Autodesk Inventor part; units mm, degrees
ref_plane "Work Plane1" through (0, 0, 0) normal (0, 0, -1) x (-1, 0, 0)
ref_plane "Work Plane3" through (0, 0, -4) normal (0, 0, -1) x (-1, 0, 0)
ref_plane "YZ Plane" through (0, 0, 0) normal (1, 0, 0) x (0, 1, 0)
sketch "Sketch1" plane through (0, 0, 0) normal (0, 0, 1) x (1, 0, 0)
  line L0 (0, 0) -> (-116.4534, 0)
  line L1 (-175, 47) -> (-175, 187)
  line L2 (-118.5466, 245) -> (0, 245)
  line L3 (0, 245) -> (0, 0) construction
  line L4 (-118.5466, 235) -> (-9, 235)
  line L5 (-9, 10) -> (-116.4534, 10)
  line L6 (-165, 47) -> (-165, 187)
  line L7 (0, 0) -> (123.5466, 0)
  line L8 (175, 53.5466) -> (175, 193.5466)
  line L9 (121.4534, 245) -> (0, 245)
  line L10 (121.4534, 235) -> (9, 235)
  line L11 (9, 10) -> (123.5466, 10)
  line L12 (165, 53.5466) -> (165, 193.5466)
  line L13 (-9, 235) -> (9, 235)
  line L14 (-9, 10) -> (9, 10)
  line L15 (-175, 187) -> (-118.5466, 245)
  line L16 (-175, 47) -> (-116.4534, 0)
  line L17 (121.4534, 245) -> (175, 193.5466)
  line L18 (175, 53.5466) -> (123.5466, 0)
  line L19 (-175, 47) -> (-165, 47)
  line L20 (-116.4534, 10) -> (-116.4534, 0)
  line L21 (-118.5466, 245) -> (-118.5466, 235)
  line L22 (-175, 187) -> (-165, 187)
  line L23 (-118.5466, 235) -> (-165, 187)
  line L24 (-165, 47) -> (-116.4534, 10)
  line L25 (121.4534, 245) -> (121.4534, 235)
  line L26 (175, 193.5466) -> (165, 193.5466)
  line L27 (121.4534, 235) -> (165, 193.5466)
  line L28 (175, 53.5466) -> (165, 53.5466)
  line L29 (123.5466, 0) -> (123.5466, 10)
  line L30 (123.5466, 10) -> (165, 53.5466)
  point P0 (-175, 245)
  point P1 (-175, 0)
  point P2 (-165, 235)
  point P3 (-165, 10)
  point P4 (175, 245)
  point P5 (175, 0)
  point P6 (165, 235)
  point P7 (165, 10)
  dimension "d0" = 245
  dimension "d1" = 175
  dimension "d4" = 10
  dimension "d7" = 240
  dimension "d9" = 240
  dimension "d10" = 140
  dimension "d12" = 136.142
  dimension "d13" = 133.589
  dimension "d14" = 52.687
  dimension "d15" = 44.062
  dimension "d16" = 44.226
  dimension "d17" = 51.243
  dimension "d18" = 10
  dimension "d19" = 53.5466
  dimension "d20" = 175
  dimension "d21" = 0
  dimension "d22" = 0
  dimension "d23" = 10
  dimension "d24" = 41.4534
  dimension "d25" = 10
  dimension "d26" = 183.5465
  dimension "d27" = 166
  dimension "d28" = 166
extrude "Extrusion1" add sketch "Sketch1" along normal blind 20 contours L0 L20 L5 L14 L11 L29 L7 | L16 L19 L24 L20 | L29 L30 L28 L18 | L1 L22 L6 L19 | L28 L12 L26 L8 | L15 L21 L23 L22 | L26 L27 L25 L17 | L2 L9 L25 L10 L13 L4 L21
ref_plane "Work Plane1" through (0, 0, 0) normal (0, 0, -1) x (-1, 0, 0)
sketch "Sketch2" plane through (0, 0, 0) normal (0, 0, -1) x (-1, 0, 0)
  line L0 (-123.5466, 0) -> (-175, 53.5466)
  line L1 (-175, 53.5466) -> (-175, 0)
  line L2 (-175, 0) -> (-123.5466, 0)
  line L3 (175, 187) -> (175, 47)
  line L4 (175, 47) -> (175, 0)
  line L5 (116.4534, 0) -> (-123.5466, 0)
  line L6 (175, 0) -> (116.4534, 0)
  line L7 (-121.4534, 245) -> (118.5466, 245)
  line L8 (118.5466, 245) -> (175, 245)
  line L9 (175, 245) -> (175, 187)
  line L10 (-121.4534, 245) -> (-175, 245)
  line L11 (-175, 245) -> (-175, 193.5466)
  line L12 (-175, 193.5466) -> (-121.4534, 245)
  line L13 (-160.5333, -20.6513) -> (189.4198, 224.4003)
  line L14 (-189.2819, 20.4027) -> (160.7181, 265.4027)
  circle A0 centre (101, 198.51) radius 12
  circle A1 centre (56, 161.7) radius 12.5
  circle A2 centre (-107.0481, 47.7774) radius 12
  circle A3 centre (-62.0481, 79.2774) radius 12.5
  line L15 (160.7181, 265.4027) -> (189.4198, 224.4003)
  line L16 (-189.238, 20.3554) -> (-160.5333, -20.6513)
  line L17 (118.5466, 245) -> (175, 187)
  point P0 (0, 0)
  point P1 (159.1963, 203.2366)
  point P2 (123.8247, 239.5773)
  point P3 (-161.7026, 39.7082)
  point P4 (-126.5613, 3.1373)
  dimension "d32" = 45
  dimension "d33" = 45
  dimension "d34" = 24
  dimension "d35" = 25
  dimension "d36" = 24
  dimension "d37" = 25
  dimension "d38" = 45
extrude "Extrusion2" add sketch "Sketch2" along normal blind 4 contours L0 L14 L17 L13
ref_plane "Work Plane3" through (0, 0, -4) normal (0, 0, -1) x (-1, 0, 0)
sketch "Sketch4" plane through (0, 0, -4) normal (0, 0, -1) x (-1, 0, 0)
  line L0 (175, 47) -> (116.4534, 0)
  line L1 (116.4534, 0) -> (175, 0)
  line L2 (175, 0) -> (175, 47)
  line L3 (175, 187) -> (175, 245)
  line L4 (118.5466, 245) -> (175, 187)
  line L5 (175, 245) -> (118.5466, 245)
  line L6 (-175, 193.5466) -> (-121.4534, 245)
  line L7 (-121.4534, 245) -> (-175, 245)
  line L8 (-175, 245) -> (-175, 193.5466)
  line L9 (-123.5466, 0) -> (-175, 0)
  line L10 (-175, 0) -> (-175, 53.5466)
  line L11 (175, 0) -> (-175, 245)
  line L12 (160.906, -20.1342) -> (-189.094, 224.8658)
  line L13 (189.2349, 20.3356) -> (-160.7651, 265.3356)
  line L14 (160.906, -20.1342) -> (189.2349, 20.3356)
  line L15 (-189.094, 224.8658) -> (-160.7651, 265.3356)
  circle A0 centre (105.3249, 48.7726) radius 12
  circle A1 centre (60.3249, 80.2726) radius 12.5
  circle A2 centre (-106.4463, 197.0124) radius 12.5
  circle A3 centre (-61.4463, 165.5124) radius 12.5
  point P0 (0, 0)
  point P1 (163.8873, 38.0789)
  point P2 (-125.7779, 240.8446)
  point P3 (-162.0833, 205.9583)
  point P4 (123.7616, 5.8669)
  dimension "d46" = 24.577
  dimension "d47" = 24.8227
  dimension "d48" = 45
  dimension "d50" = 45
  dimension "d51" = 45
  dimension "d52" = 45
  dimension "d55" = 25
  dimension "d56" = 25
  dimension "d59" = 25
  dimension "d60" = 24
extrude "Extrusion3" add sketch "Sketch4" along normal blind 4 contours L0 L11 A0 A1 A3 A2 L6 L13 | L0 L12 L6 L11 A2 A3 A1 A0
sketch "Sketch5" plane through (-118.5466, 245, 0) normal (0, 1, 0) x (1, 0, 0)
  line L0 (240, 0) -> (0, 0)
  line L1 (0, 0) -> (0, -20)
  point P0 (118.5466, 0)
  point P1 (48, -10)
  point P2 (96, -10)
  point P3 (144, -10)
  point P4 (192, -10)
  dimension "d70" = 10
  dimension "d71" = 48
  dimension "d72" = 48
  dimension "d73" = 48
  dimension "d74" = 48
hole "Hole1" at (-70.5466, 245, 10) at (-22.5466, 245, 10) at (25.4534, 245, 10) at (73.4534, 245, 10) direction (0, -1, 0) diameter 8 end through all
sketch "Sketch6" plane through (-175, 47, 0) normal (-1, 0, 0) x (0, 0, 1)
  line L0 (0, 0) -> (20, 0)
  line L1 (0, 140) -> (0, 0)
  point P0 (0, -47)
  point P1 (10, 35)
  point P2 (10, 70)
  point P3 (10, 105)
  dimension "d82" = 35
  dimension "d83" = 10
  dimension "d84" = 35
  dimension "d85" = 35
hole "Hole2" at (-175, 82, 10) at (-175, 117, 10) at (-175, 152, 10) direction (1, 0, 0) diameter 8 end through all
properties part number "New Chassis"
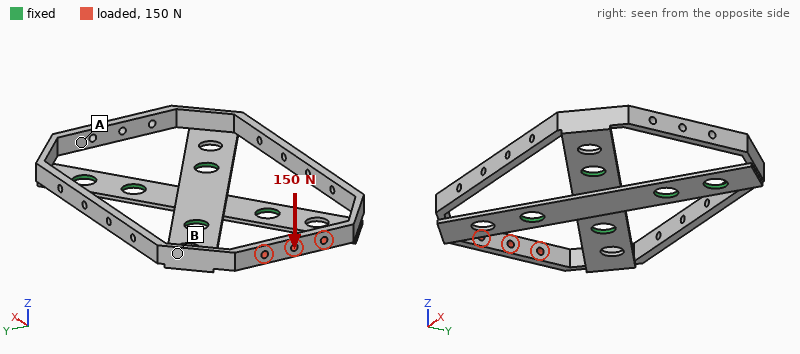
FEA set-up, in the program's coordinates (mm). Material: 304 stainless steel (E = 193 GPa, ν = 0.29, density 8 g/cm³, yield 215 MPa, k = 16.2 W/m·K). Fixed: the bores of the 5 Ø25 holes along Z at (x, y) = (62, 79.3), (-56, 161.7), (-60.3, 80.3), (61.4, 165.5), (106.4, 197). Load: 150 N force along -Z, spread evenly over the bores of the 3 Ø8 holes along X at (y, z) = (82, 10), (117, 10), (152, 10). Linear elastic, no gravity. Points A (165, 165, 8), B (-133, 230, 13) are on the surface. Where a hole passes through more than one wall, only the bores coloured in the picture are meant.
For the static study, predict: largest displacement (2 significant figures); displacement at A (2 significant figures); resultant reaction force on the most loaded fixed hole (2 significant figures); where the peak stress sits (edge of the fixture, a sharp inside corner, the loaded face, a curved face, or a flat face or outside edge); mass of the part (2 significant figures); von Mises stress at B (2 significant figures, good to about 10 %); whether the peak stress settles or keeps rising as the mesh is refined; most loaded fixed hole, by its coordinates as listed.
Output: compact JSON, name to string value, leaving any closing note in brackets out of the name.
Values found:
{"largest displacement": "1.6 mm", "displacement at A": "1.1 mm", "resultant reaction force on the most loaded fixed hole": "150 N", "where the peak stress sits": "edge of the fixture", "mass of the part": "2.5 kg", "von Mises stress at B": "11 MPa", "whether the peak stress settles or keeps rising as the mesh is refined": "keeps rising", "most loaded fixed hole, by its coordinates as listed": "(-56, 161.7)"}
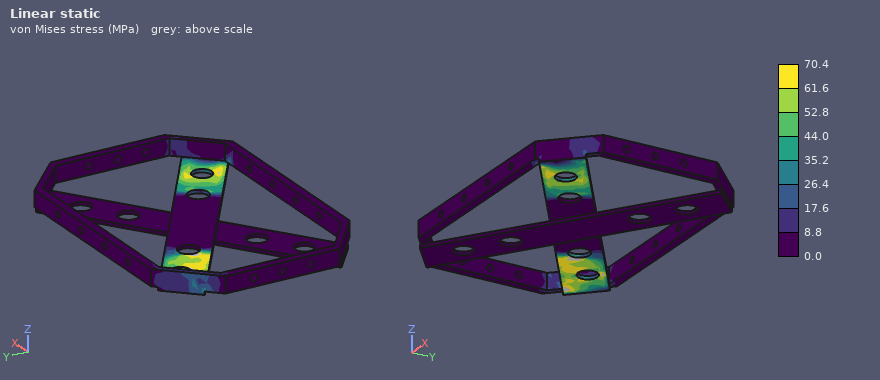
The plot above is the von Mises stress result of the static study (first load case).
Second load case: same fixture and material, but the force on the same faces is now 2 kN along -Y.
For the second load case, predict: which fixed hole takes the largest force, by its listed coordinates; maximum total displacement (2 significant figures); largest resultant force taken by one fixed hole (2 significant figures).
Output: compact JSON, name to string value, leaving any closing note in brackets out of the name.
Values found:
{"which fixed hole takes the largest force, by its listed coordinates": "(-56, 161.7)", "maximum total displacement": "1.8 mm", "largest resultant force taken by one fixed hole": "2.4 kN"}
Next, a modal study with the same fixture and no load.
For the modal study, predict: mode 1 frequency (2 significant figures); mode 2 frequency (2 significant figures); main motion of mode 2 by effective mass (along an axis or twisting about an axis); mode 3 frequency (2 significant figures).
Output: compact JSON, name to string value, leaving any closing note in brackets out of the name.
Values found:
{"mode 1 frequency": "52 Hz", "mode 2 frequency": "150 Hz", "main motion of mode 2 by effective mass": "along Z", "mode 3 frequency": "190 Hz"}
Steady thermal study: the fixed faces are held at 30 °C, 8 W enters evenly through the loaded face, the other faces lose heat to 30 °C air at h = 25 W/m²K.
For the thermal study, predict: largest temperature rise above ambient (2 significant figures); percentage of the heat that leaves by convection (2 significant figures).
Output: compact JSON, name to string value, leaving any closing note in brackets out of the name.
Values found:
{"largest temperature rise above ambient": "40 K", "percentage of the heat that leaves by convection": "100 %"}
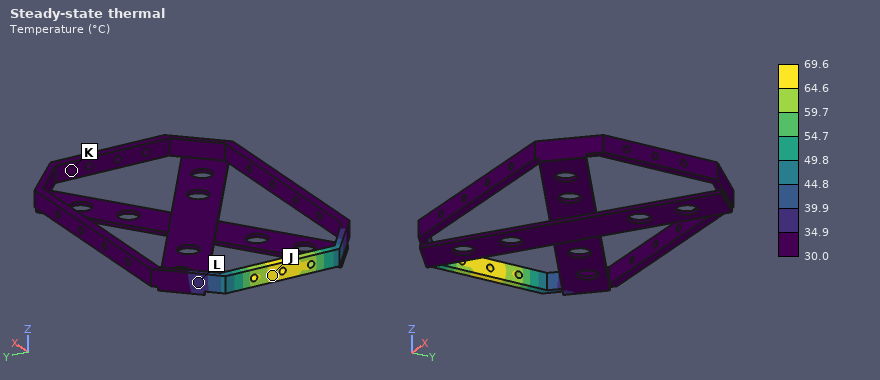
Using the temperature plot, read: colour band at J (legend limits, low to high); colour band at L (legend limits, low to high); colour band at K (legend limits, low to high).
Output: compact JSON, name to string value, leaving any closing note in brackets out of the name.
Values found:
{"colour band at J": "64.6 to 69.6 °C", "colour band at L": "34.9 to 39.9 °C", "colour band at K": "30.0 to 34.9 °C"}
